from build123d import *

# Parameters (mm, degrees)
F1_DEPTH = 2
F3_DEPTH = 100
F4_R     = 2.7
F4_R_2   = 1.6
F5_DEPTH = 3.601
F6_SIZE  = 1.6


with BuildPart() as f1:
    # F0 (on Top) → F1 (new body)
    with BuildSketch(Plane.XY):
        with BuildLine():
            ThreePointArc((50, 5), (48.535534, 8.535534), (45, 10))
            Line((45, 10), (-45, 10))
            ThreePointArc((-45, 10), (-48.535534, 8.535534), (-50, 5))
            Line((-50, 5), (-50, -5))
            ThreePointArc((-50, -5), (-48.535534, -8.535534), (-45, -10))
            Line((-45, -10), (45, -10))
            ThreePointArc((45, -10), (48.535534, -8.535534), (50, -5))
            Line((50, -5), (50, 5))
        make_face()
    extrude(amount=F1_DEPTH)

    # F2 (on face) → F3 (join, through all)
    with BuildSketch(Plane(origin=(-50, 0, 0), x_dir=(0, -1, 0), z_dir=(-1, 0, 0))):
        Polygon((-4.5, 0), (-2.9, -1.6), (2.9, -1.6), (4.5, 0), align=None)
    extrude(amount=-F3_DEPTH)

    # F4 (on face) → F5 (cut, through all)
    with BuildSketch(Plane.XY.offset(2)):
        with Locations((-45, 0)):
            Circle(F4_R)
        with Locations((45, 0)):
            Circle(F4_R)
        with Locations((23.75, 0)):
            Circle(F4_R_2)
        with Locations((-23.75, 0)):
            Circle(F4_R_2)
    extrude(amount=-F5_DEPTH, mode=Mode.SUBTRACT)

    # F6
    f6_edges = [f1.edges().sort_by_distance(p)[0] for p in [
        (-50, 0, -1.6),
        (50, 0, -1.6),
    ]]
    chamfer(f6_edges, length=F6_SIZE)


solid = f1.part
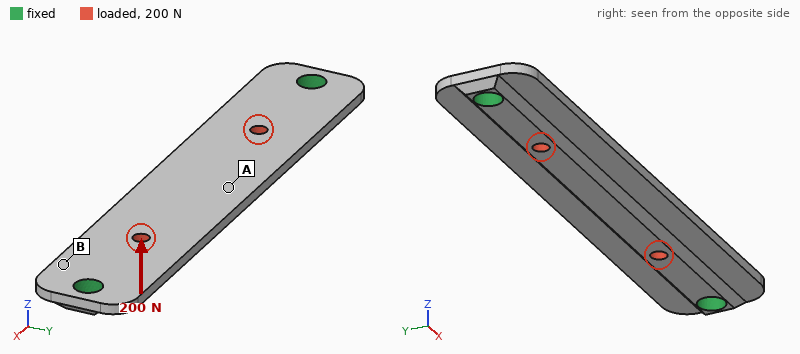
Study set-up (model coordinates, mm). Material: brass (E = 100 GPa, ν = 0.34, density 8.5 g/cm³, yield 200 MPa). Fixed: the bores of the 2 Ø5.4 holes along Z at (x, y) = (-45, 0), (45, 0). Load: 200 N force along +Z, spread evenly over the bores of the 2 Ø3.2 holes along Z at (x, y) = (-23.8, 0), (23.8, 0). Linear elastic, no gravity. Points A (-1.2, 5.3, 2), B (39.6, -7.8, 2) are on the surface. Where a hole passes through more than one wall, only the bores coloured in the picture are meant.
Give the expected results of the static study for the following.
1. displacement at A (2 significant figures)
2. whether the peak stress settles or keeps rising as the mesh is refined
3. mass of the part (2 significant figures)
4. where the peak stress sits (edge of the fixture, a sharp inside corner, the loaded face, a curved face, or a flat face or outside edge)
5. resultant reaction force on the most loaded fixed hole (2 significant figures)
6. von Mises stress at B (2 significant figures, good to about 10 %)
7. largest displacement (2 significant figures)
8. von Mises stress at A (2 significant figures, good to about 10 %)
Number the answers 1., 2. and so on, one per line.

1. 67 µm
2. keeps rising
3. 42 g
4. edge of the fixture
5. 110 N
6. 28 MPa
7. 69 µm
8. 14 MPa
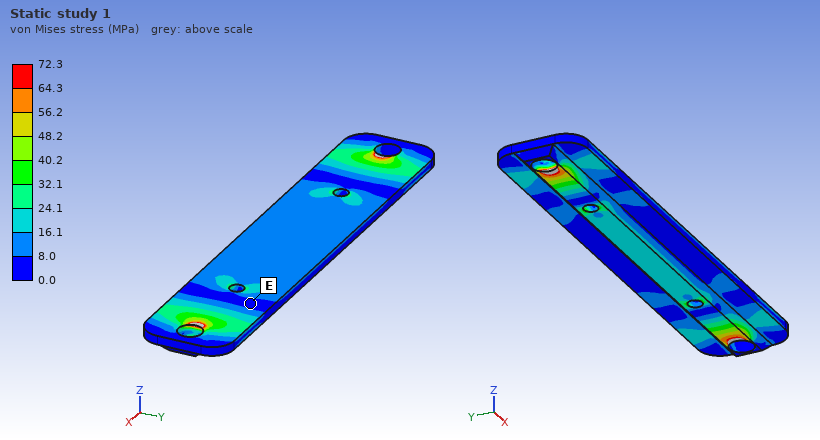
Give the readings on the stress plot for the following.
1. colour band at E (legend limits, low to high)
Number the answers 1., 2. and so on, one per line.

1. 0.0 to 8.0 MPa
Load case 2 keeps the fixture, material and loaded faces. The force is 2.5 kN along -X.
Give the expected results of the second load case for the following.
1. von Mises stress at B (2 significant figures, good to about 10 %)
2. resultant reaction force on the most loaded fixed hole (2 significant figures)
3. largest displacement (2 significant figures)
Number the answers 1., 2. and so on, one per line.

1. 14 MPa
2. 1.3 kN
3. 7.5 µm
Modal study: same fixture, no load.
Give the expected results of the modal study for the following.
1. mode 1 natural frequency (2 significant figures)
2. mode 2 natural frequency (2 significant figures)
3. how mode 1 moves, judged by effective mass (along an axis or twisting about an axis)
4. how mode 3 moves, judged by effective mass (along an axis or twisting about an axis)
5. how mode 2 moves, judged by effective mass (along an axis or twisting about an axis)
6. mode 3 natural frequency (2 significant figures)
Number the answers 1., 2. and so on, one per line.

1. 1500 Hz
2. 3600 Hz
3. along Z
4. twisting about Y
5. twisting about X
6. 3900 Hz
